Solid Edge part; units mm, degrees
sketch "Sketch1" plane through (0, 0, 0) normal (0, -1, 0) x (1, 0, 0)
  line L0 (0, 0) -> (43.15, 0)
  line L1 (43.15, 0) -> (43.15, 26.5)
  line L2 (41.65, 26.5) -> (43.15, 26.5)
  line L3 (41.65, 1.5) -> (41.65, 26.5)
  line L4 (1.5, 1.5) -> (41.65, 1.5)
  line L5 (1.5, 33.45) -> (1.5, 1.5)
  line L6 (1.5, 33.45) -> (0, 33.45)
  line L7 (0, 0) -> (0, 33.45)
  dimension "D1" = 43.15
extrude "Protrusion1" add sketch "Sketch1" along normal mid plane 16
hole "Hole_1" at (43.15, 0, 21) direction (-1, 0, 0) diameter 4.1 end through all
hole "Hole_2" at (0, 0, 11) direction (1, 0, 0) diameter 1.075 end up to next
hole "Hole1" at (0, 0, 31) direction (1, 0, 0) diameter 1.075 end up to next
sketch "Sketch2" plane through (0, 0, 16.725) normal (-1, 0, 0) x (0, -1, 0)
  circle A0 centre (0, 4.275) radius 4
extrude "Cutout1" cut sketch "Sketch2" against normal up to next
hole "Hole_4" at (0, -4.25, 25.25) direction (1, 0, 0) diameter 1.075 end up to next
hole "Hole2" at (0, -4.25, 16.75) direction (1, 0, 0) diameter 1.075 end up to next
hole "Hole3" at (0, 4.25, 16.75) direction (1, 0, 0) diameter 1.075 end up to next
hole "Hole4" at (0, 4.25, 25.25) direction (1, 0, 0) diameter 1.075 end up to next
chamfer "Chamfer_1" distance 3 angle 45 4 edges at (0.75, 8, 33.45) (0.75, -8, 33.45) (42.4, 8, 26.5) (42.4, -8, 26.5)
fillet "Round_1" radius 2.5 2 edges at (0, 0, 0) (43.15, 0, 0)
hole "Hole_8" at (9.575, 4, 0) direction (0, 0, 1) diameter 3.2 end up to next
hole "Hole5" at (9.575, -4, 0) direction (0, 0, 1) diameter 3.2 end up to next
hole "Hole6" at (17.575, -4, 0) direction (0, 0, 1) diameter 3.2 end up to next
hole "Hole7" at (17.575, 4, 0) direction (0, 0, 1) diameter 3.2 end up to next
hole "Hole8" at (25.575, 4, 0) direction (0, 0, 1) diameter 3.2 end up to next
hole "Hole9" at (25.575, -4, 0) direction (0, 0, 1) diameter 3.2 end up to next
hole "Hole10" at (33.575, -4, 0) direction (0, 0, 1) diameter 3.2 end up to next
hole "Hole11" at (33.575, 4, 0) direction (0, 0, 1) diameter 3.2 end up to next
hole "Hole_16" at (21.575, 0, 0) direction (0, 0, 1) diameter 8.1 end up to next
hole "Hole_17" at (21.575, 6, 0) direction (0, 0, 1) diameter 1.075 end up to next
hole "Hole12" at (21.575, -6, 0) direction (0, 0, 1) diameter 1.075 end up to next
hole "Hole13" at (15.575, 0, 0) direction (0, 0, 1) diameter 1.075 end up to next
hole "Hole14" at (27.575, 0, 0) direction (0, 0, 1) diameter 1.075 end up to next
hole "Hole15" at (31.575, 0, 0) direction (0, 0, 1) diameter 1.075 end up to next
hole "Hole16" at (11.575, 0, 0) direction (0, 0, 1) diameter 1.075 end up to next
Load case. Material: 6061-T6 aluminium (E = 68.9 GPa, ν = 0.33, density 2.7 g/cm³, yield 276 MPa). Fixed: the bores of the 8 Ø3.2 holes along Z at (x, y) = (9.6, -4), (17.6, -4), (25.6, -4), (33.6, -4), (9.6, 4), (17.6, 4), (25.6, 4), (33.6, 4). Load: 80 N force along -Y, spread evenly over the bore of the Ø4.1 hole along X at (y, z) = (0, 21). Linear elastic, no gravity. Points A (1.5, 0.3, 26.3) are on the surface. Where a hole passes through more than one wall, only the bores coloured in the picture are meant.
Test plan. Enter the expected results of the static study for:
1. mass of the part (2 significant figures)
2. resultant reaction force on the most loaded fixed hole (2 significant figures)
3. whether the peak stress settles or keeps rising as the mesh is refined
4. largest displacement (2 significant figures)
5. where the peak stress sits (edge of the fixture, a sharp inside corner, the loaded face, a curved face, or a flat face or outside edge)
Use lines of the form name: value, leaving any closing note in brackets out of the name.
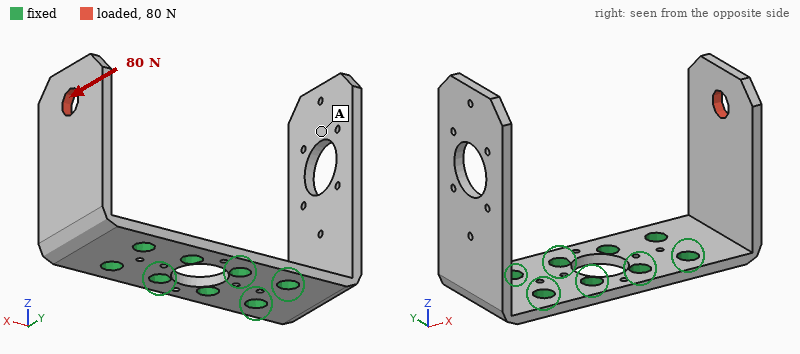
mass of the part: 5.5 g
resultant reaction force on the most loaded fixed hole: 170 N
whether the peak stress settles or keeps rising as the mesh is refined: keeps rising
largest displacement: 0.34 mm
where the peak stress sits: edge of the fixture
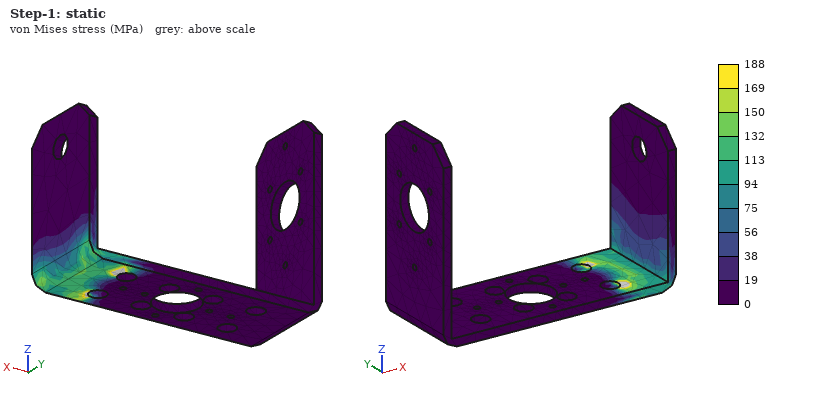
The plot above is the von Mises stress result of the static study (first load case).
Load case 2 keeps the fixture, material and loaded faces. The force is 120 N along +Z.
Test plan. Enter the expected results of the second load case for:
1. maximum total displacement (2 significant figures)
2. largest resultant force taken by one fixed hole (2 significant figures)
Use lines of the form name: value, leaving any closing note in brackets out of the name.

maximum total displacement: 0.29 mm
largest resultant force taken by one fixed hole: 62 N
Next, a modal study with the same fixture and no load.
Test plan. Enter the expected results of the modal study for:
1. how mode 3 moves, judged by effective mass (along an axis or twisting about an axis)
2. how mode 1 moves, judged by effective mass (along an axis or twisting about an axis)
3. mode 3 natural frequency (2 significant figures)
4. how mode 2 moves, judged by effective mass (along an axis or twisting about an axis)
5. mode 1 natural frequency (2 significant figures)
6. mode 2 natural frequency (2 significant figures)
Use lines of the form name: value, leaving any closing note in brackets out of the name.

how mode 3 moves, judged by effective mass: along Y
how mode 1 moves, judged by effective mass: along X
mode 3 natural frequency: 2200 Hz
how mode 2 moves, judged by effective mass: along X
mode 1 natural frequency: 910 Hz
mode 2 natural frequency: 1400 Hz
